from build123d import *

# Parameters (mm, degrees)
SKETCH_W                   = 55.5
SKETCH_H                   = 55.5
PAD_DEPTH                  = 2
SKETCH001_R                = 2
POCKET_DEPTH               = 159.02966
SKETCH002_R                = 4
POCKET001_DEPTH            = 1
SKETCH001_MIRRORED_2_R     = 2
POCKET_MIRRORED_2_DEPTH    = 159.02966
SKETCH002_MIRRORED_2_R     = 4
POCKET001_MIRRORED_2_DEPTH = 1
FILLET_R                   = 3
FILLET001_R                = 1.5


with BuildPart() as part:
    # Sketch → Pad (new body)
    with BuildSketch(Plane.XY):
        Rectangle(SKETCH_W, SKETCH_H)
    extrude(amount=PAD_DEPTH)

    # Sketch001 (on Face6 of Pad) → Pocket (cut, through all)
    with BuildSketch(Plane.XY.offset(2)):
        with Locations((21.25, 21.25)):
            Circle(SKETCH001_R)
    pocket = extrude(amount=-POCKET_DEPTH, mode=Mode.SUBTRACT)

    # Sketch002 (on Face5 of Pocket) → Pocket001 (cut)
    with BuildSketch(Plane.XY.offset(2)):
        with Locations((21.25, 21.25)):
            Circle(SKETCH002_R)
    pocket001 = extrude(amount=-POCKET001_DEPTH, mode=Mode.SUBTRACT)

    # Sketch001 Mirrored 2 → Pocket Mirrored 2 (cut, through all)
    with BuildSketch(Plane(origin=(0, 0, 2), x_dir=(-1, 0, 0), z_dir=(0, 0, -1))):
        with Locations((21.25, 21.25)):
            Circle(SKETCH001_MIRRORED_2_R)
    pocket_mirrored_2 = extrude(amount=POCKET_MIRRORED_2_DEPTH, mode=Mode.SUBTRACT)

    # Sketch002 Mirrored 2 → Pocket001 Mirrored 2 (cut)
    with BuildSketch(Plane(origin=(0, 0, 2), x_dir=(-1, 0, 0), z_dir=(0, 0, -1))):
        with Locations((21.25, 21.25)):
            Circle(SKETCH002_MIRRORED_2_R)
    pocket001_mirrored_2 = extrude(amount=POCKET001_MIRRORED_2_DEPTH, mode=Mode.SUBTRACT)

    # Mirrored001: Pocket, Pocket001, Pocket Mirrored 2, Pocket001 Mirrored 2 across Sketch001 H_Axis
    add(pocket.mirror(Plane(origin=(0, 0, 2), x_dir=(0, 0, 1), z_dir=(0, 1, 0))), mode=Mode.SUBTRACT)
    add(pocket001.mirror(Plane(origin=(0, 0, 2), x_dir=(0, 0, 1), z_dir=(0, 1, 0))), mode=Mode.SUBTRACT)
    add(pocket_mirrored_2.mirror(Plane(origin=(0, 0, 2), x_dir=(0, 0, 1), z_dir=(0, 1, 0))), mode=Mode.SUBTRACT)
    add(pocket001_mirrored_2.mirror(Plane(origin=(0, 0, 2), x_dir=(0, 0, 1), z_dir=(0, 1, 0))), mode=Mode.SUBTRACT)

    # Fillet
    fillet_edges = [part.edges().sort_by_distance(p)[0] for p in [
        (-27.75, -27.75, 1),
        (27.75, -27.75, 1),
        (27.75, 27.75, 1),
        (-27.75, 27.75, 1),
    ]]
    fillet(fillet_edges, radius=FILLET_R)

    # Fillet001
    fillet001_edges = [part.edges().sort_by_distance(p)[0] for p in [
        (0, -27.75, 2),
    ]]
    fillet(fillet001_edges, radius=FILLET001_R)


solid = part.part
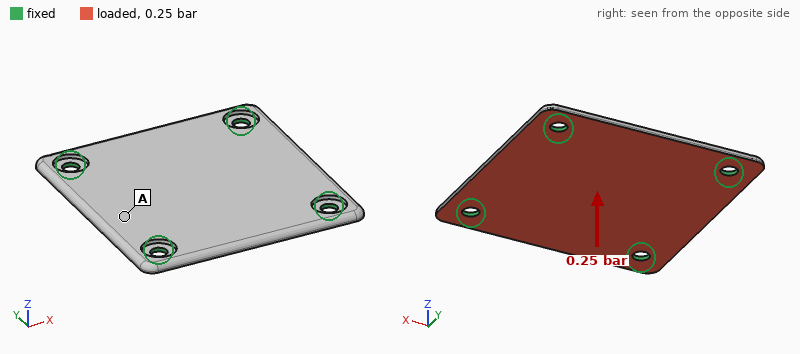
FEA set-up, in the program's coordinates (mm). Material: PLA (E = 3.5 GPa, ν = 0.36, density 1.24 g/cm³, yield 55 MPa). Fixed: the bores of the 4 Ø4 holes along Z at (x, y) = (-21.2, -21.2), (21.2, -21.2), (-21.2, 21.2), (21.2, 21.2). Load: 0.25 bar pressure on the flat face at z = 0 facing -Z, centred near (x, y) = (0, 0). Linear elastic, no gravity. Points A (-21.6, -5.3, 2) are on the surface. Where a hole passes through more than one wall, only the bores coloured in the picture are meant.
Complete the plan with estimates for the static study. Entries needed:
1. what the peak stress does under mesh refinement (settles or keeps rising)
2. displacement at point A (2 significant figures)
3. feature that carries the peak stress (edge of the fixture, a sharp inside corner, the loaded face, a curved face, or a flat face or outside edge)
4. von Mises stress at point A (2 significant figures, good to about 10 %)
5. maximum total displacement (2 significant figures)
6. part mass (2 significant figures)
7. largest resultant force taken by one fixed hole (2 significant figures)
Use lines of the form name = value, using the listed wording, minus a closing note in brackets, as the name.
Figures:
what the peak stress does under mesh refinement = keeps rising
displacement at point A = 0.14 mm
feature that carries the peak stress = edge of the fixture
von Mises stress at point A = 4.0 MPa
maximum total displacement = 0.26 mm
part mass = 7.2 g
largest resultant force taken by one fixed hole = 37 N
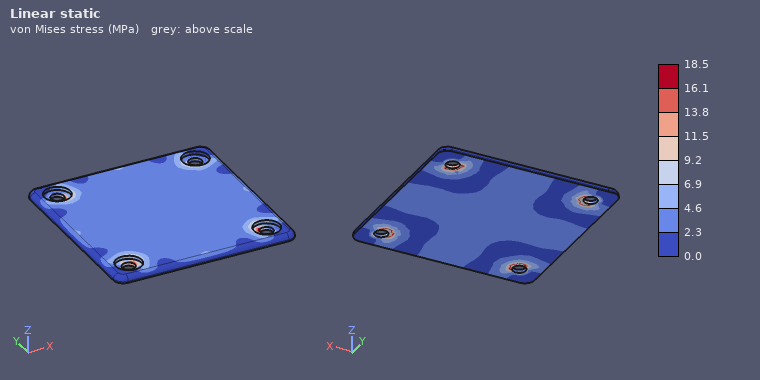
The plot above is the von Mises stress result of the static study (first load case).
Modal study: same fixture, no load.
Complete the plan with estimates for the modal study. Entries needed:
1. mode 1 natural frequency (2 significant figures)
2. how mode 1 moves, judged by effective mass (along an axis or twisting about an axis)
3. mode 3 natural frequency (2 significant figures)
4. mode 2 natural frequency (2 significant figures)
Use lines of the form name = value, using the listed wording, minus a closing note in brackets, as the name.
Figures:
mode 1 natural frequency = 1200 Hz
how mode 1 moves, judged by effective mass = along Z
mode 3 natural frequency = 1900 Hz
mode 2 natural frequency = 1900 Hz
